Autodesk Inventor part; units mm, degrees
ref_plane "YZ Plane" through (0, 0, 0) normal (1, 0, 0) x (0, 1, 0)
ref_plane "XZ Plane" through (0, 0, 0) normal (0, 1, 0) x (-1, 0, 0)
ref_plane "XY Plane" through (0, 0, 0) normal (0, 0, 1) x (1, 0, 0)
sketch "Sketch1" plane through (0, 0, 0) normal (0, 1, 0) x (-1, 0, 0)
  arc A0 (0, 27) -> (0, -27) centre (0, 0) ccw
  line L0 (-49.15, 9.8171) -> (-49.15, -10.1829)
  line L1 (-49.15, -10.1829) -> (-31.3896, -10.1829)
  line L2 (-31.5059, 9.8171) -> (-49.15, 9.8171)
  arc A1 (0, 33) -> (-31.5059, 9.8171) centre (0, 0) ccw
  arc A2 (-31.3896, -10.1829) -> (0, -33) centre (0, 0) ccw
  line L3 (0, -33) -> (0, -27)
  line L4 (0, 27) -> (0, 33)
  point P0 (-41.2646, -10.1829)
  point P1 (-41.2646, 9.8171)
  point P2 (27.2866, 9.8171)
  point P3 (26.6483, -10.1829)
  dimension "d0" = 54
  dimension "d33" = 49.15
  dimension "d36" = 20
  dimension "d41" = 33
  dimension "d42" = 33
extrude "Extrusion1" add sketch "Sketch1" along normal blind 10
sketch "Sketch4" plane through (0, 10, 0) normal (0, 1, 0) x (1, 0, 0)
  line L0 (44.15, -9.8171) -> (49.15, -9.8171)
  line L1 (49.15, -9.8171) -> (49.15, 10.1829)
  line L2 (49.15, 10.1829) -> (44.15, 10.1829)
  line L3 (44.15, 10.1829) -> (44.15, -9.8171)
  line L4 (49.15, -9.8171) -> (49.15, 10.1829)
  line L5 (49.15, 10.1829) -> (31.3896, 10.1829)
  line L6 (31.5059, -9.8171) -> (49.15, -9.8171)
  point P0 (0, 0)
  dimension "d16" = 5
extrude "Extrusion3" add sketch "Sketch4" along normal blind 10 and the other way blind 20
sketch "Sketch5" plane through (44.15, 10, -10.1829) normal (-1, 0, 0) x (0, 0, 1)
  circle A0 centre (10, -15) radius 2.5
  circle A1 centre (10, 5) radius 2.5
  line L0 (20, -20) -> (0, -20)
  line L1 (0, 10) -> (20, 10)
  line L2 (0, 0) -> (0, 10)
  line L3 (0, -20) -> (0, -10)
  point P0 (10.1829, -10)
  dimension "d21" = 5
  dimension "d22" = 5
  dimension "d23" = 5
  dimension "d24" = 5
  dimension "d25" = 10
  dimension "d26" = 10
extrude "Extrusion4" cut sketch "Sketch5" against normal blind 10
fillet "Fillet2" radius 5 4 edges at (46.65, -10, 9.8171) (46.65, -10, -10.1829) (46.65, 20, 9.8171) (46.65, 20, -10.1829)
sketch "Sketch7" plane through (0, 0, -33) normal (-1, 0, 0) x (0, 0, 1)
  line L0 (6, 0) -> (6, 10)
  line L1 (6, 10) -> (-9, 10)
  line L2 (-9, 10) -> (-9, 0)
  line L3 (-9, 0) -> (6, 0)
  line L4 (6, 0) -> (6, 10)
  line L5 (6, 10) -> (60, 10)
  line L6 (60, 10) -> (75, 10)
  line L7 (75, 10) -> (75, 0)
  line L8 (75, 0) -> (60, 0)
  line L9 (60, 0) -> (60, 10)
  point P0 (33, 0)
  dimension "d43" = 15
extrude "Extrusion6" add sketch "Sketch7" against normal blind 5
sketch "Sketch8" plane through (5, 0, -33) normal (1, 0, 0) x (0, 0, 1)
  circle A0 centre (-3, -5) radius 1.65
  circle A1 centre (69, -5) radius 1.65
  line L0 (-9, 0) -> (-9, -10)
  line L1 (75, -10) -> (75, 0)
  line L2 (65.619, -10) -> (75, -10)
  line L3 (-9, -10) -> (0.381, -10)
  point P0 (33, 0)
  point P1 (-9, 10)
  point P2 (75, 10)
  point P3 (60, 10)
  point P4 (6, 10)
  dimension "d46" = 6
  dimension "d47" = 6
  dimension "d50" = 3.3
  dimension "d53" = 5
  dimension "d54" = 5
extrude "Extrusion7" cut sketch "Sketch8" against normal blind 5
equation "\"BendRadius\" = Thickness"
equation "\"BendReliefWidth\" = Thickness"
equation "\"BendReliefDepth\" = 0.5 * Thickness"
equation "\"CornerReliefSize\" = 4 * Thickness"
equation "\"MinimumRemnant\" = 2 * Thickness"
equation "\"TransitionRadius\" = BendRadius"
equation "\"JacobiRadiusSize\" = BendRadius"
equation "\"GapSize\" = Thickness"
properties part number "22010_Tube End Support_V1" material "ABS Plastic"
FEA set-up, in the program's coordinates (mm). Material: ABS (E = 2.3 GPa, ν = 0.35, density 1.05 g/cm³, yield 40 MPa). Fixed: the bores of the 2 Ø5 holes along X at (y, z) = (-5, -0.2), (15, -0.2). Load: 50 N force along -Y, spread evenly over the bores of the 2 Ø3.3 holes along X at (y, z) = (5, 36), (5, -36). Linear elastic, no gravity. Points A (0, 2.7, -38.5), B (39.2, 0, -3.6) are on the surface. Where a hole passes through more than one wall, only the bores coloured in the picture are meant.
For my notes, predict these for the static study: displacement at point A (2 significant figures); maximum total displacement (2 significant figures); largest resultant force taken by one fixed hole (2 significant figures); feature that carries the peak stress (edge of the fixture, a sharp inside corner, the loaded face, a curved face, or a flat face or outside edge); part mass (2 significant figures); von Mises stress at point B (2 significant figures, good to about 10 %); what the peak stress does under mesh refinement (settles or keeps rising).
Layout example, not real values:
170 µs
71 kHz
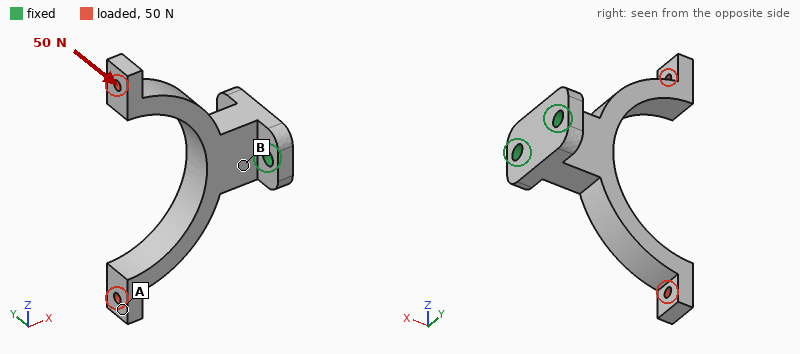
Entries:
1.1 mm
1.1 mm
140 N
a sharp inside corner
12 g
5.2 MPa
keeps rising
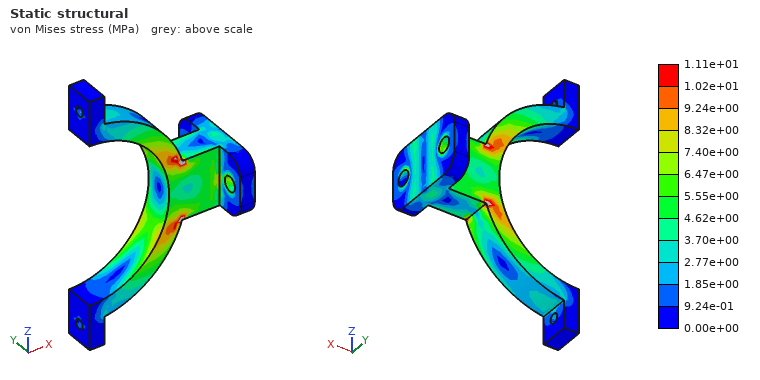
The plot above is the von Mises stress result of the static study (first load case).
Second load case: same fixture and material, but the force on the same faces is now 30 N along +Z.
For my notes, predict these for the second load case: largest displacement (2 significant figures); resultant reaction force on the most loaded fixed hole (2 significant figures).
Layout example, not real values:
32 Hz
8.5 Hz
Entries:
1.1 mm
15 N
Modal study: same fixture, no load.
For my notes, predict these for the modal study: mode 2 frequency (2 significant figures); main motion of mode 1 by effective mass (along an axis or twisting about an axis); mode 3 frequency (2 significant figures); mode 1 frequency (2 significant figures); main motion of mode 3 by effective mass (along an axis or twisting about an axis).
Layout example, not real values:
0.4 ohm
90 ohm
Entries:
650 Hz
along Z
720 Hz
500 Hz
along Y
